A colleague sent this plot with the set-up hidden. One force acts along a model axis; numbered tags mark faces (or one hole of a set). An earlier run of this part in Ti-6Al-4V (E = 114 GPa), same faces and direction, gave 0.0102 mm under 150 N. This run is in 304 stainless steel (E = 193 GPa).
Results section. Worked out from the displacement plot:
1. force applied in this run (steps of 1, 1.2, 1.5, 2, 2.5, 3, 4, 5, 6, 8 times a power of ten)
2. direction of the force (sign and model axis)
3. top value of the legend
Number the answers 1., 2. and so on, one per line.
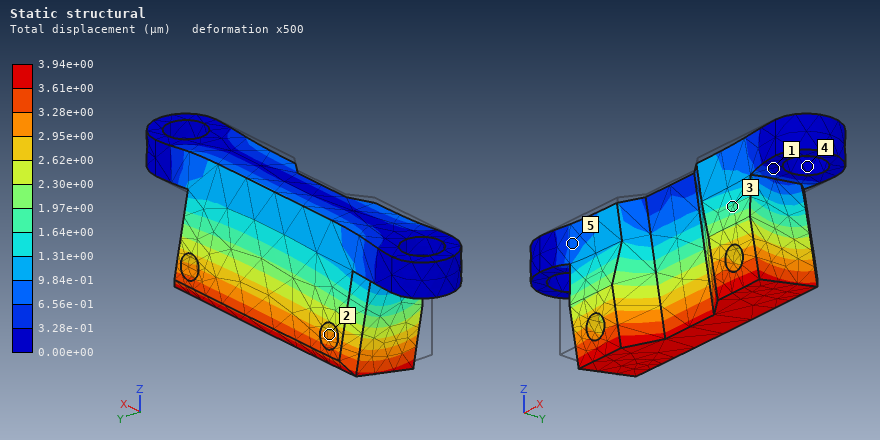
1. 100 N
2. +Y
3. 3.94e+00 µm
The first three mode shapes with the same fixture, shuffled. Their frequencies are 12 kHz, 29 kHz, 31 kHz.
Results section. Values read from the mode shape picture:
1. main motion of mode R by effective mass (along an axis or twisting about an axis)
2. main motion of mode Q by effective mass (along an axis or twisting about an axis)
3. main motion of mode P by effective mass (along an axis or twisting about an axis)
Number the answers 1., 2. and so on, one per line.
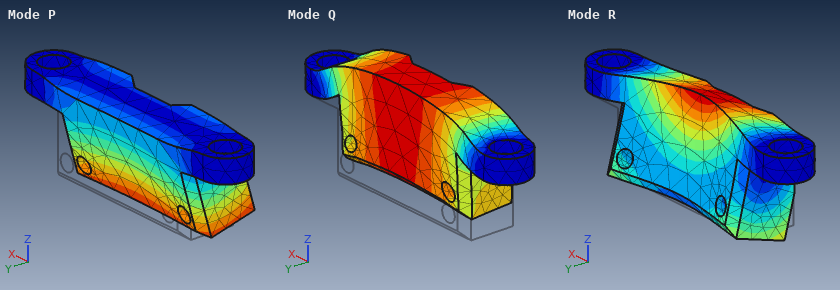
1. along Y
2. along Z
3. along Y
